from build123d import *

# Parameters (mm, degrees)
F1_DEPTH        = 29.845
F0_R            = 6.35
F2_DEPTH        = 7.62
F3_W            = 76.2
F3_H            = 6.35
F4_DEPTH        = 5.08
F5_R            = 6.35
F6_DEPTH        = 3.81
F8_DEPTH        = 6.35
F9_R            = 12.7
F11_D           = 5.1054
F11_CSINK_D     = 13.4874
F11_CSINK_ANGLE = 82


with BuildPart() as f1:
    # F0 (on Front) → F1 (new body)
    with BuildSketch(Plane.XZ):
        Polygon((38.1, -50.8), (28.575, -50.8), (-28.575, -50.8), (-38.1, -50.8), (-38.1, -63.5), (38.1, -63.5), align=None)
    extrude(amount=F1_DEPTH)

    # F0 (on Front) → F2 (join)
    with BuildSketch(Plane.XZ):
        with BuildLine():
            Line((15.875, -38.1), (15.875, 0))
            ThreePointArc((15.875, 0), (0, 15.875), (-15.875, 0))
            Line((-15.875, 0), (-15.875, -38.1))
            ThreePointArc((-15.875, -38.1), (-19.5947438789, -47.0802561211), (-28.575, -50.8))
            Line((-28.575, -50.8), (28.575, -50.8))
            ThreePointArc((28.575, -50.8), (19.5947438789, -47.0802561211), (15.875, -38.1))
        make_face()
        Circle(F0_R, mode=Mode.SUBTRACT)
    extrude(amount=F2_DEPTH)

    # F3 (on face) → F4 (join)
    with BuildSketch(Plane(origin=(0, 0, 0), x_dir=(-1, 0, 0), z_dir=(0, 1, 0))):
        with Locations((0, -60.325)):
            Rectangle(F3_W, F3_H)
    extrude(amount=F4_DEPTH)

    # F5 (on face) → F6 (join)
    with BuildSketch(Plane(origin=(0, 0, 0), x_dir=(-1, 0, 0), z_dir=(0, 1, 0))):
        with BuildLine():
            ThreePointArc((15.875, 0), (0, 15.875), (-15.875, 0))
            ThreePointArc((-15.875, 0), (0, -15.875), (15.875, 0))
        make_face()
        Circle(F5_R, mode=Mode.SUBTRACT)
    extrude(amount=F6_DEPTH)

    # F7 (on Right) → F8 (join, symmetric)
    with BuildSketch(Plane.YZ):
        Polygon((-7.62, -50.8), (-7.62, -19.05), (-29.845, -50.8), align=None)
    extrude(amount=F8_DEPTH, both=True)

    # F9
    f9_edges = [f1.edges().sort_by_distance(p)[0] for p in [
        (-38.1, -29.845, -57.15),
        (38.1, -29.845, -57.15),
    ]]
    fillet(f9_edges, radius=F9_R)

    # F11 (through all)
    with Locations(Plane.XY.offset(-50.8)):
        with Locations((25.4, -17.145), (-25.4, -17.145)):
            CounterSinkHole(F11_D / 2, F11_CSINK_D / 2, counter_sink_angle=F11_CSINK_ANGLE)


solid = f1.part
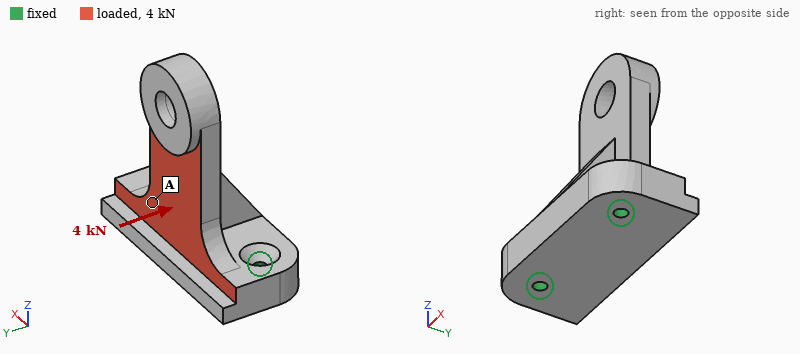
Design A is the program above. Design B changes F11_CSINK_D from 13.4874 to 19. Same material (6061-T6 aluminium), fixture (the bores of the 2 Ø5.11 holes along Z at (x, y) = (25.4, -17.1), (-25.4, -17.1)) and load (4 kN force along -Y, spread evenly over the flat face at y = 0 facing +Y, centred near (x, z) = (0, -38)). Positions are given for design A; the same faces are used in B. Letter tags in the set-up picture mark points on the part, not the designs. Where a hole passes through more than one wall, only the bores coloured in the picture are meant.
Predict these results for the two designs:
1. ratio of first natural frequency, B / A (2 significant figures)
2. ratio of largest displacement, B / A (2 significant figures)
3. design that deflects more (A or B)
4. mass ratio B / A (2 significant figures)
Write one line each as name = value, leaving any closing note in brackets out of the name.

ratio of first natural frequency, B / A = 0.77
ratio of largest displacement, B / A = 2.0
design that deflects more = B
mass ratio B / A = 0.98
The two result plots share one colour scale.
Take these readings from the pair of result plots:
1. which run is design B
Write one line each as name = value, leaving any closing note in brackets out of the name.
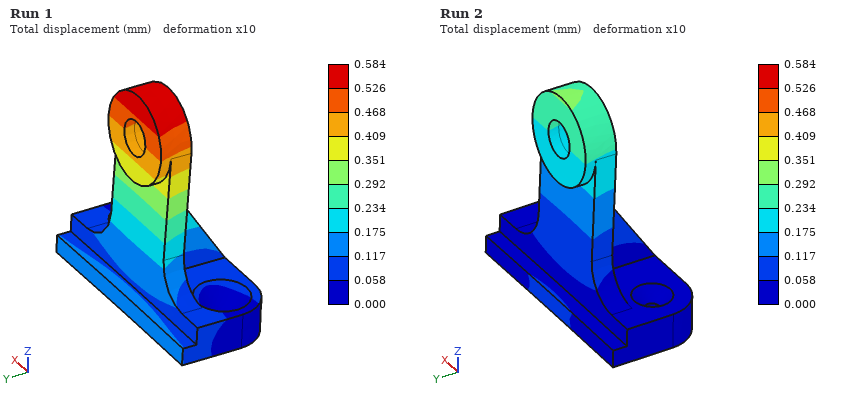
which run is design B = Run 1
